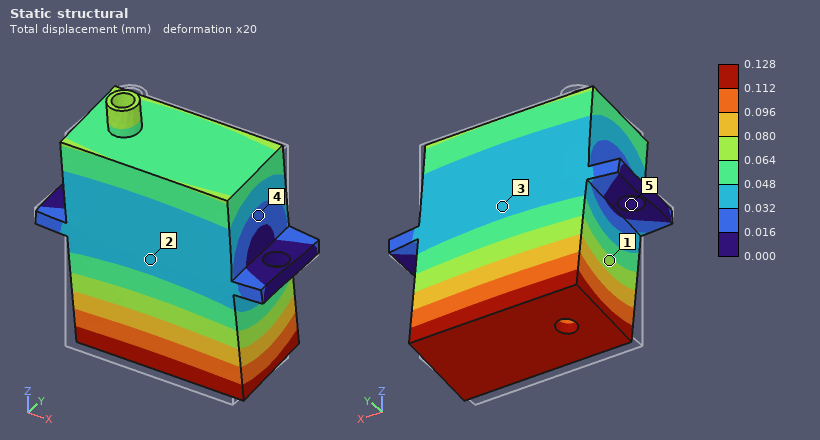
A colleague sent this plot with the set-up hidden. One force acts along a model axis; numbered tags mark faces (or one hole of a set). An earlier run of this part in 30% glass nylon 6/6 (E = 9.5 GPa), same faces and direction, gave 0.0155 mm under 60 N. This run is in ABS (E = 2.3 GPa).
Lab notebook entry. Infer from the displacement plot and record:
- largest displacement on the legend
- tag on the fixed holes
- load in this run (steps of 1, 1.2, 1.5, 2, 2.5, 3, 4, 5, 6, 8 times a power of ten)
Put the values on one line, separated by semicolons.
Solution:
0.128 mm; 5; 120 N
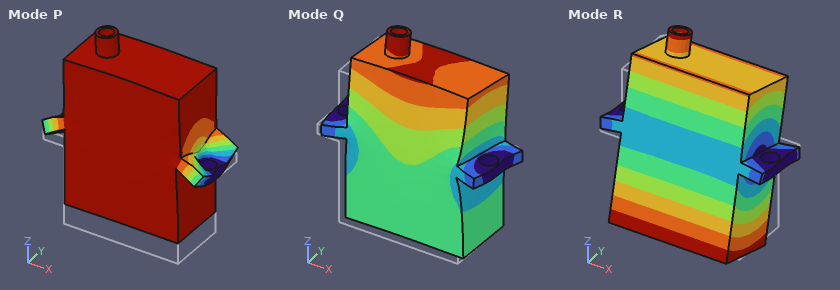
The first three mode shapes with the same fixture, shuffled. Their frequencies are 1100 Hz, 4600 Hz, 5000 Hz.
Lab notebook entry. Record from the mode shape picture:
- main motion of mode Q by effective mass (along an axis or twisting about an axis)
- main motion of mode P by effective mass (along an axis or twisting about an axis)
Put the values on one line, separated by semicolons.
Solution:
along Y; along Z
